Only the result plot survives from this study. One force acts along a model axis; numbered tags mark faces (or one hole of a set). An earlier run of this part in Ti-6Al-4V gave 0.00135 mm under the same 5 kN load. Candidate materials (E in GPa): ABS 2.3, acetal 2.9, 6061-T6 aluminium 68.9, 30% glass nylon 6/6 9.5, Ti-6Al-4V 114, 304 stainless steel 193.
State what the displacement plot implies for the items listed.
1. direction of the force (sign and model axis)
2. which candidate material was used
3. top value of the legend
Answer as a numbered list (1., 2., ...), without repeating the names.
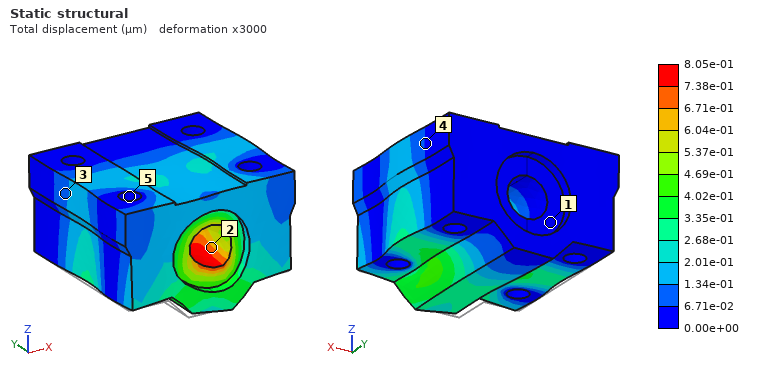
1. +X
2. 304 stainless steel
3. 8.05e-01 µm
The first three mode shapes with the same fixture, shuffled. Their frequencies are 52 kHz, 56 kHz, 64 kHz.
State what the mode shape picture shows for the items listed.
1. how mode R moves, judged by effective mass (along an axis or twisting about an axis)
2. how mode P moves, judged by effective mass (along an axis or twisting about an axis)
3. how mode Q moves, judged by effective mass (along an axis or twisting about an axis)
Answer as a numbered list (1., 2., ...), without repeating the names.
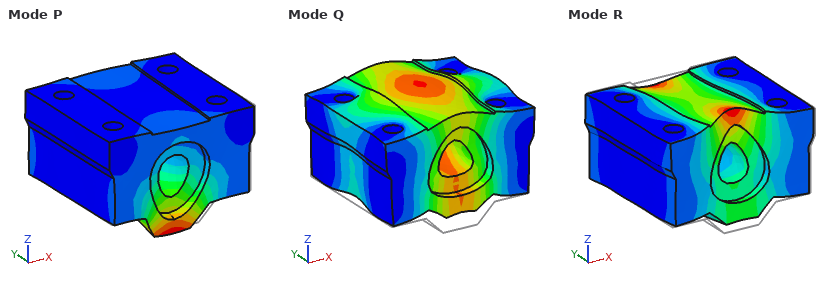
1. along Y
2. along Y
3. along Z
